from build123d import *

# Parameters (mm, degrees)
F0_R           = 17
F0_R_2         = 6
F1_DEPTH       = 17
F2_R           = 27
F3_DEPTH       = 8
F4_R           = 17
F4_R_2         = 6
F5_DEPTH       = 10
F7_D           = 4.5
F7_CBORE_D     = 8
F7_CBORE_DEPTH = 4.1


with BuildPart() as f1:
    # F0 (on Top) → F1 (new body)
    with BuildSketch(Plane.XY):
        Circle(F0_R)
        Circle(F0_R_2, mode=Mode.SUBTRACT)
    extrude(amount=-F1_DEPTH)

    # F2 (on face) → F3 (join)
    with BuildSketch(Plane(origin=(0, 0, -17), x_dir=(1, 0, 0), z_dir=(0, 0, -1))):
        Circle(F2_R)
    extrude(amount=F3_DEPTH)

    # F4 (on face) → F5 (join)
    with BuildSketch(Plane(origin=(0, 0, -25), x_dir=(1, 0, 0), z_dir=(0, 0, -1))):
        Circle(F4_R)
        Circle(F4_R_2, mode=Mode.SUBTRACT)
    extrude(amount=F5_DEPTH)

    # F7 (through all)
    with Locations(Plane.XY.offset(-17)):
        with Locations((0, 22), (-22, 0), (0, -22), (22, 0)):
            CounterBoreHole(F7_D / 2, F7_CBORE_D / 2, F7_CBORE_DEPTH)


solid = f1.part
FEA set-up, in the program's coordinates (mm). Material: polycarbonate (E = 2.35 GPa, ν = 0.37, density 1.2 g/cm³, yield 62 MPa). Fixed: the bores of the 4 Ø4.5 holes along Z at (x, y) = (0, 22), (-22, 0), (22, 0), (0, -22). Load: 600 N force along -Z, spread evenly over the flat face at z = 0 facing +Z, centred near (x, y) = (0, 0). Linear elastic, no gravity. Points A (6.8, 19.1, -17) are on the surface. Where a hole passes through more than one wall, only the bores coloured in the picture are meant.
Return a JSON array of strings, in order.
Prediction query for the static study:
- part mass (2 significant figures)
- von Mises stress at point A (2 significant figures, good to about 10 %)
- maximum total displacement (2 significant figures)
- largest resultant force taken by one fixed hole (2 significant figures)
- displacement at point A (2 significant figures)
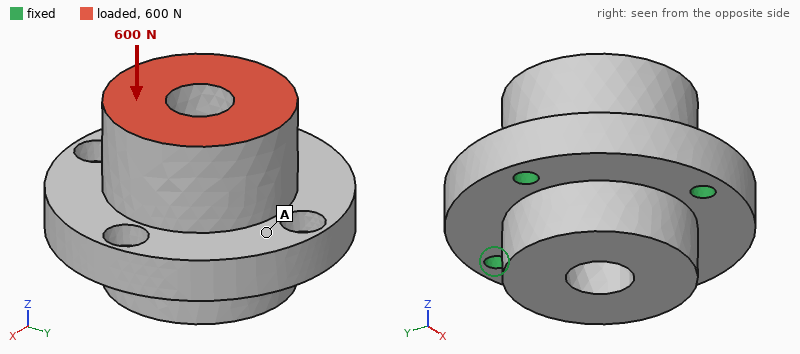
["46 g", "1.1 MPa", "25 µm", "160 N", "14 µm"]
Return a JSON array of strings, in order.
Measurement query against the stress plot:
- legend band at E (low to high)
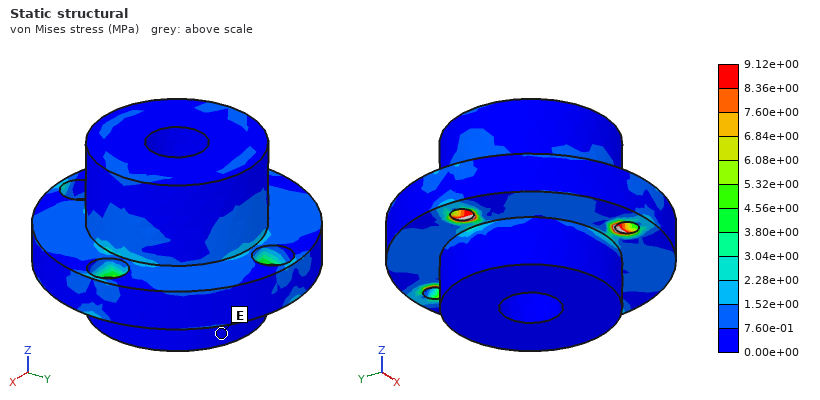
["0.00e+00 to 7.60e-01 MPa"]
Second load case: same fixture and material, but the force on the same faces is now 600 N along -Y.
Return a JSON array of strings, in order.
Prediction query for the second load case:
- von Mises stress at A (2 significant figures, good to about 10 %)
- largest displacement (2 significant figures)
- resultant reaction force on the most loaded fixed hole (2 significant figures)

["3.5 MPa", "97 µm", "390 N"]
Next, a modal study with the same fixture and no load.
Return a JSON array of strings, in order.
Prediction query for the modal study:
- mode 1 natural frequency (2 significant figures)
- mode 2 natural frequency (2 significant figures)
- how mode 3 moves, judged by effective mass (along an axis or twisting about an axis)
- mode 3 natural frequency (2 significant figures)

["4100 Hz", "4100 Hz", "along Z", "4300 Hz"]
